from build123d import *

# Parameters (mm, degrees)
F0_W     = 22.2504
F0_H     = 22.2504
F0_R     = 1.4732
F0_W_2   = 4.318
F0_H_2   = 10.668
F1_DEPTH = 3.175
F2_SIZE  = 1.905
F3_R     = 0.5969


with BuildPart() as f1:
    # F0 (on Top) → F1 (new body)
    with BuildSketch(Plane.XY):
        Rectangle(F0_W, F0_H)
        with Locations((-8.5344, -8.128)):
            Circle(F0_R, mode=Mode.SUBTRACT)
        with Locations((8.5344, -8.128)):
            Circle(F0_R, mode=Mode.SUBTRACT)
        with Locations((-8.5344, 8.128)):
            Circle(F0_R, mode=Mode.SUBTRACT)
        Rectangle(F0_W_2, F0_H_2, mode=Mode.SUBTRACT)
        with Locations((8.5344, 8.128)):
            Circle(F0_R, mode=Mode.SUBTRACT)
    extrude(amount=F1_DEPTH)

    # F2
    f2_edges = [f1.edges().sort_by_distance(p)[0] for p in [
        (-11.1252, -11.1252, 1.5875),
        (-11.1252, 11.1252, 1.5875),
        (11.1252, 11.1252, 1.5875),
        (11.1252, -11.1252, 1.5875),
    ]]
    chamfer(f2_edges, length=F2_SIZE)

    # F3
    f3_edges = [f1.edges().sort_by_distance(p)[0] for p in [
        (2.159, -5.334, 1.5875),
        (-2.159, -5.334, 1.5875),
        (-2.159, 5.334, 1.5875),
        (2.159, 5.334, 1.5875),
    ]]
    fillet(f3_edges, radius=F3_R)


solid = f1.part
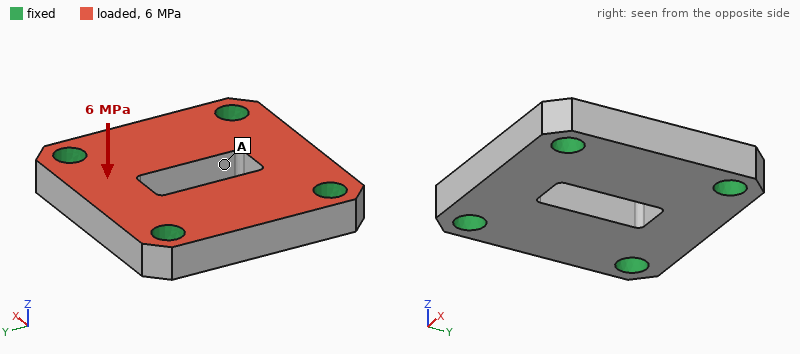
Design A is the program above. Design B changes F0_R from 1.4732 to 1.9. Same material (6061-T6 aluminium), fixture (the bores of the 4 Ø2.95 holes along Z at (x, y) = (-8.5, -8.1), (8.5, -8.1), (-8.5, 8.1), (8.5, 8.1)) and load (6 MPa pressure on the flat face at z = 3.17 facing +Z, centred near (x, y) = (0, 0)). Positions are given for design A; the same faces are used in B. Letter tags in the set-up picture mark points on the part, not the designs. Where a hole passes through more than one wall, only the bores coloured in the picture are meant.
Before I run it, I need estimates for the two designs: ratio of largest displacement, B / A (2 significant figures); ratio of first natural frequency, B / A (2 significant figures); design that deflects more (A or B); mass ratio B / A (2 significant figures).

0.79
1.1
A
0.96
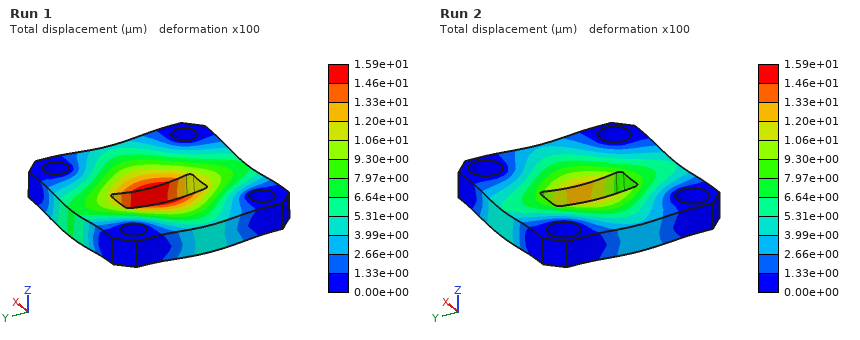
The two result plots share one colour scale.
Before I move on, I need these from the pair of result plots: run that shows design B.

Run 2
